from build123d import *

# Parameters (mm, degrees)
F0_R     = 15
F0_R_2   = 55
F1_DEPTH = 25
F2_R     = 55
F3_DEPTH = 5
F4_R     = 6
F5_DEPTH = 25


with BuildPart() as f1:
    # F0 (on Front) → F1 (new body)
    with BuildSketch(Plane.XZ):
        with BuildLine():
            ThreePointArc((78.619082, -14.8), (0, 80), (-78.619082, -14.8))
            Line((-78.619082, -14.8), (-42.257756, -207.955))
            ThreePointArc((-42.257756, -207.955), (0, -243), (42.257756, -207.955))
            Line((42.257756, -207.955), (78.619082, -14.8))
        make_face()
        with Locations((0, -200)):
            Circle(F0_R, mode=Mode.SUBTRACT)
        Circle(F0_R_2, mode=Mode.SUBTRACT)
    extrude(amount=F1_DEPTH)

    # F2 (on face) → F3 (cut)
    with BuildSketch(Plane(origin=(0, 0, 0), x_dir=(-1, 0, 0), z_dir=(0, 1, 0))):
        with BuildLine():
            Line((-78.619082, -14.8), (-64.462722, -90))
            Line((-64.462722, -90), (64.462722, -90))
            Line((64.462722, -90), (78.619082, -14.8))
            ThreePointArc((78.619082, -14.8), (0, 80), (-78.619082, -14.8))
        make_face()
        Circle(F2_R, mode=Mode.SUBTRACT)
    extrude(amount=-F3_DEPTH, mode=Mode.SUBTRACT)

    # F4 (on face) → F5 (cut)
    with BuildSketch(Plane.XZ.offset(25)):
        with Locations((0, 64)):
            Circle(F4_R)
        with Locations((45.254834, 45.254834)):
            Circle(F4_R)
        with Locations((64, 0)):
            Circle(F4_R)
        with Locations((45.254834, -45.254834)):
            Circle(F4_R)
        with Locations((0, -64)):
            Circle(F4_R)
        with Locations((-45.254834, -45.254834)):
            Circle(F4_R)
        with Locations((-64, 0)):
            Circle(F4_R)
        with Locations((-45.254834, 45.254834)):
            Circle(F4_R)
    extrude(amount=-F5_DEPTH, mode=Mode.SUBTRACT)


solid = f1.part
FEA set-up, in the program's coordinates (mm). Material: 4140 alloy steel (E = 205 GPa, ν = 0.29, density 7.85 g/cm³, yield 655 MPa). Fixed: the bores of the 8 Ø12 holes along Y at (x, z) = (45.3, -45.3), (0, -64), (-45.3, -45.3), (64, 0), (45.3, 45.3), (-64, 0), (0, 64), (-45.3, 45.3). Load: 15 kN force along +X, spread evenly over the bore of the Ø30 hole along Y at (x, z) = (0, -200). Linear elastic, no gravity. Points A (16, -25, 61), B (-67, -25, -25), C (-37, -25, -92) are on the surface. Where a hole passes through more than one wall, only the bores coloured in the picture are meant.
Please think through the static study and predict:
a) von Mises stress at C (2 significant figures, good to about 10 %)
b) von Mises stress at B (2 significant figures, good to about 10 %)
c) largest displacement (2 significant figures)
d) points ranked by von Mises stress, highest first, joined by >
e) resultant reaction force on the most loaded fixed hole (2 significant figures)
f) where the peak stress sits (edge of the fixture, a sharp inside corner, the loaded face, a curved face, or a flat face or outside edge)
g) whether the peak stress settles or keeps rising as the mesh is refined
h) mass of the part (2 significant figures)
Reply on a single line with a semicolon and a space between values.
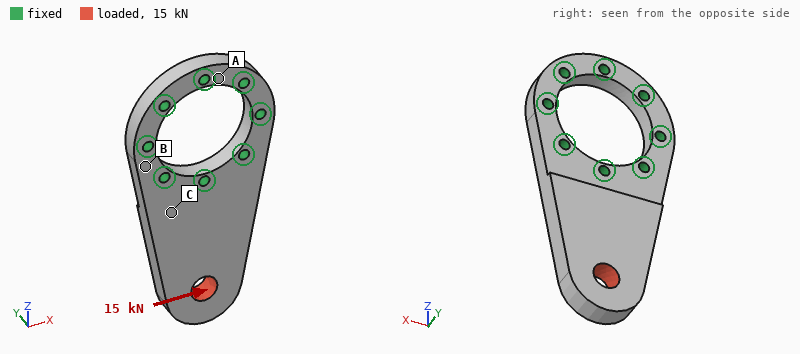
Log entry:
19 MPa; 11 MPa; 50 µm; C > B > A; 17 kN; edge of the fixture; keeps rising; 4.8 kg
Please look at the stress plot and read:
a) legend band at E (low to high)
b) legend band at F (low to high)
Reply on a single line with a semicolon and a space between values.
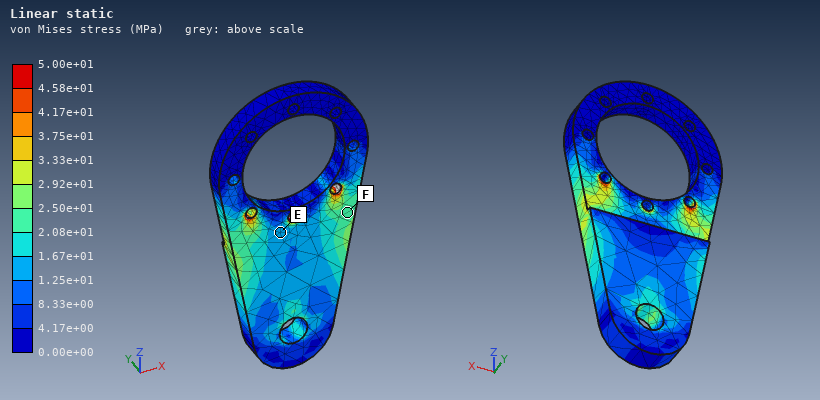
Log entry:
1.25e+01 to 1.67e+01 MPa; 2.08e+01 to 2.50e+01 MPa
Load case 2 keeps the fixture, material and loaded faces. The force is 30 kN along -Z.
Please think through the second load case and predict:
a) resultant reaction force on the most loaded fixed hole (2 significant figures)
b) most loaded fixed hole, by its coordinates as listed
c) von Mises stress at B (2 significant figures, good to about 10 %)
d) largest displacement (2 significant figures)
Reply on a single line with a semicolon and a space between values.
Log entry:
12 kN; (0, -64); 3.2 MPa; 29 µm
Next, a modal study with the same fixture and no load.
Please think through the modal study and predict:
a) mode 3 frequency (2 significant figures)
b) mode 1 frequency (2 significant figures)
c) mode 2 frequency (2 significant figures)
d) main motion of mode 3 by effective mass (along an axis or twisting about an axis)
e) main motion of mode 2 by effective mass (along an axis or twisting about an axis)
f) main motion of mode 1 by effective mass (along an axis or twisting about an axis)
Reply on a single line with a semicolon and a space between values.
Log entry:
2700 Hz; 640 Hz; 2400 Hz; along X; twisting about Z; along Y
